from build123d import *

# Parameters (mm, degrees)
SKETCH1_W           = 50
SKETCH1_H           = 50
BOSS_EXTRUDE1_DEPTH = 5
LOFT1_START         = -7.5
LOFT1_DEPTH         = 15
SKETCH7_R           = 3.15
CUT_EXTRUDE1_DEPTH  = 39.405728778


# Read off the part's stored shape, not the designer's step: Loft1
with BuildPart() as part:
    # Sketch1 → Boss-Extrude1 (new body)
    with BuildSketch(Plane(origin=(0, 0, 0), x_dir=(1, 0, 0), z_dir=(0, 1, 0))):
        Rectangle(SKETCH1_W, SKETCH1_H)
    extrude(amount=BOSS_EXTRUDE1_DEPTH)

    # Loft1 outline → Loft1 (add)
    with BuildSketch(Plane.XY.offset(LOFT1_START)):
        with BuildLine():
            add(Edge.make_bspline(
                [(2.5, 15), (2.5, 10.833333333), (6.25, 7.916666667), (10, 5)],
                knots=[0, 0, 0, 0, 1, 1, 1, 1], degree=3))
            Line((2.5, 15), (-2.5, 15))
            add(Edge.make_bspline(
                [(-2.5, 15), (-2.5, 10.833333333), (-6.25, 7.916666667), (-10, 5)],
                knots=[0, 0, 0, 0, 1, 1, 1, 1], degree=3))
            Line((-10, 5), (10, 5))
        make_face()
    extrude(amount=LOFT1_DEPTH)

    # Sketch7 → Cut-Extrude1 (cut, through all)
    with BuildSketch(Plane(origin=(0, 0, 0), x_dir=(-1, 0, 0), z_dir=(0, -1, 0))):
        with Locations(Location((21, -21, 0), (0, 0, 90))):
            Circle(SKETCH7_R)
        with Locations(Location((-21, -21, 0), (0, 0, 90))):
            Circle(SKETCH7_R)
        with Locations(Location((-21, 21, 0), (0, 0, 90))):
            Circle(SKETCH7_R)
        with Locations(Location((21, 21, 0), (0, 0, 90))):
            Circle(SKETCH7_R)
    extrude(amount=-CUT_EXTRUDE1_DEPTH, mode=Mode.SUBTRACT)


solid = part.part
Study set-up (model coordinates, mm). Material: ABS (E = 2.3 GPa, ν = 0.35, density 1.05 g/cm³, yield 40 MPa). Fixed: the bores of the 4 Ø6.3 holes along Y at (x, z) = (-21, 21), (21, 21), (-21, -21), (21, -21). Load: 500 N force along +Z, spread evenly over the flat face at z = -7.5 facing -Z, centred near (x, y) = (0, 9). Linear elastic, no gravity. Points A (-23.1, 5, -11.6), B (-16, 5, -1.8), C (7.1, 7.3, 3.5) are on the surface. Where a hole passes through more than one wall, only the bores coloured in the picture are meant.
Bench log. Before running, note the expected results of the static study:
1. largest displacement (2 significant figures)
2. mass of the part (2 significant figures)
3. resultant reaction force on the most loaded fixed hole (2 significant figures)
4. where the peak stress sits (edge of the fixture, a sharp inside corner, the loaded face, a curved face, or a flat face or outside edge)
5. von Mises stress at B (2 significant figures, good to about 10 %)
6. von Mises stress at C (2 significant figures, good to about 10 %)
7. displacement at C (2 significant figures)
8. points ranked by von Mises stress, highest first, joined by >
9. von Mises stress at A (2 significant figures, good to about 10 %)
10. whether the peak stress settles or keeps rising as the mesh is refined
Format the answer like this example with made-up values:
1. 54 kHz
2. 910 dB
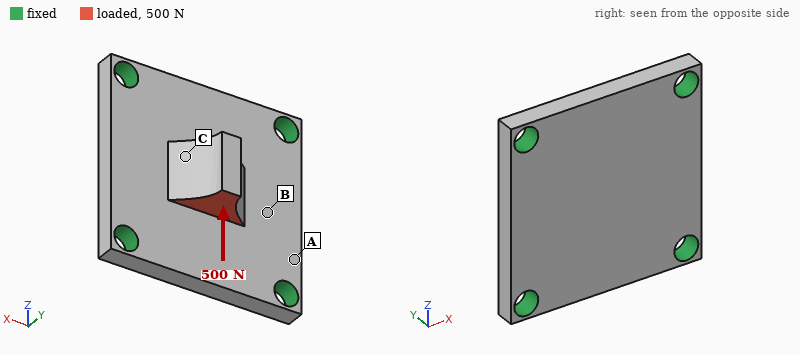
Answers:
1. 0.15 mm
2. 14 g
3. 150 N
4. edge of the fixture
5. 3.3 MPa
6. 5.3 MPa
7. 0.056 mm
8. C > B > A
9. 1.4 MPa
10. keeps rising
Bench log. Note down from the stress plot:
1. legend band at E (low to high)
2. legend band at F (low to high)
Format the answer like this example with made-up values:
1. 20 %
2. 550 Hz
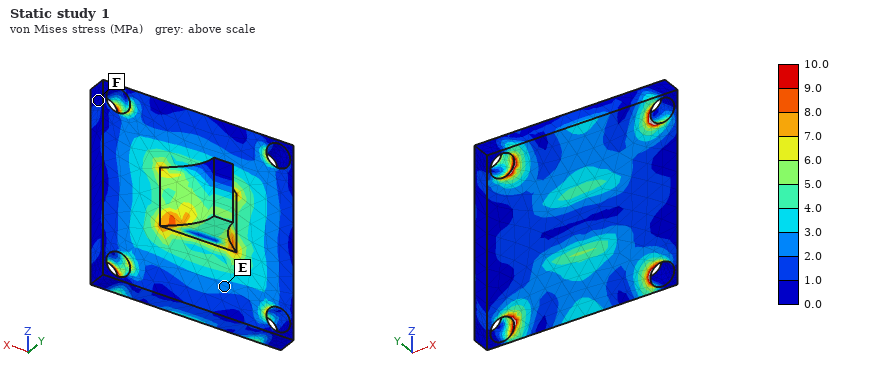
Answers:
1. 2.0 to 3.0 MPa
2. 0.0 to 1.0 MPa
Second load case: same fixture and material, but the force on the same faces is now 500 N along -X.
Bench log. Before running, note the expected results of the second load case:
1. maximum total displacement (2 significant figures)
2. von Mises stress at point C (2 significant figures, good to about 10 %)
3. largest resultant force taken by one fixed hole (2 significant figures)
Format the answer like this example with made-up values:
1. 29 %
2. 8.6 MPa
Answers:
1. 0.17 mm
2. 5.3 MPa
3. 170 N
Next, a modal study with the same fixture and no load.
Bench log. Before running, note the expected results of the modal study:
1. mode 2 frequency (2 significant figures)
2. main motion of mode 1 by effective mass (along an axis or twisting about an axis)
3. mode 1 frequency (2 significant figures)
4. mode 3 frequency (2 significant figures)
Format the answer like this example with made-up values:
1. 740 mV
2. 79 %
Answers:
1. 4900 Hz
2. along Y
3. 3000 Hz
4. 4900 Hz
